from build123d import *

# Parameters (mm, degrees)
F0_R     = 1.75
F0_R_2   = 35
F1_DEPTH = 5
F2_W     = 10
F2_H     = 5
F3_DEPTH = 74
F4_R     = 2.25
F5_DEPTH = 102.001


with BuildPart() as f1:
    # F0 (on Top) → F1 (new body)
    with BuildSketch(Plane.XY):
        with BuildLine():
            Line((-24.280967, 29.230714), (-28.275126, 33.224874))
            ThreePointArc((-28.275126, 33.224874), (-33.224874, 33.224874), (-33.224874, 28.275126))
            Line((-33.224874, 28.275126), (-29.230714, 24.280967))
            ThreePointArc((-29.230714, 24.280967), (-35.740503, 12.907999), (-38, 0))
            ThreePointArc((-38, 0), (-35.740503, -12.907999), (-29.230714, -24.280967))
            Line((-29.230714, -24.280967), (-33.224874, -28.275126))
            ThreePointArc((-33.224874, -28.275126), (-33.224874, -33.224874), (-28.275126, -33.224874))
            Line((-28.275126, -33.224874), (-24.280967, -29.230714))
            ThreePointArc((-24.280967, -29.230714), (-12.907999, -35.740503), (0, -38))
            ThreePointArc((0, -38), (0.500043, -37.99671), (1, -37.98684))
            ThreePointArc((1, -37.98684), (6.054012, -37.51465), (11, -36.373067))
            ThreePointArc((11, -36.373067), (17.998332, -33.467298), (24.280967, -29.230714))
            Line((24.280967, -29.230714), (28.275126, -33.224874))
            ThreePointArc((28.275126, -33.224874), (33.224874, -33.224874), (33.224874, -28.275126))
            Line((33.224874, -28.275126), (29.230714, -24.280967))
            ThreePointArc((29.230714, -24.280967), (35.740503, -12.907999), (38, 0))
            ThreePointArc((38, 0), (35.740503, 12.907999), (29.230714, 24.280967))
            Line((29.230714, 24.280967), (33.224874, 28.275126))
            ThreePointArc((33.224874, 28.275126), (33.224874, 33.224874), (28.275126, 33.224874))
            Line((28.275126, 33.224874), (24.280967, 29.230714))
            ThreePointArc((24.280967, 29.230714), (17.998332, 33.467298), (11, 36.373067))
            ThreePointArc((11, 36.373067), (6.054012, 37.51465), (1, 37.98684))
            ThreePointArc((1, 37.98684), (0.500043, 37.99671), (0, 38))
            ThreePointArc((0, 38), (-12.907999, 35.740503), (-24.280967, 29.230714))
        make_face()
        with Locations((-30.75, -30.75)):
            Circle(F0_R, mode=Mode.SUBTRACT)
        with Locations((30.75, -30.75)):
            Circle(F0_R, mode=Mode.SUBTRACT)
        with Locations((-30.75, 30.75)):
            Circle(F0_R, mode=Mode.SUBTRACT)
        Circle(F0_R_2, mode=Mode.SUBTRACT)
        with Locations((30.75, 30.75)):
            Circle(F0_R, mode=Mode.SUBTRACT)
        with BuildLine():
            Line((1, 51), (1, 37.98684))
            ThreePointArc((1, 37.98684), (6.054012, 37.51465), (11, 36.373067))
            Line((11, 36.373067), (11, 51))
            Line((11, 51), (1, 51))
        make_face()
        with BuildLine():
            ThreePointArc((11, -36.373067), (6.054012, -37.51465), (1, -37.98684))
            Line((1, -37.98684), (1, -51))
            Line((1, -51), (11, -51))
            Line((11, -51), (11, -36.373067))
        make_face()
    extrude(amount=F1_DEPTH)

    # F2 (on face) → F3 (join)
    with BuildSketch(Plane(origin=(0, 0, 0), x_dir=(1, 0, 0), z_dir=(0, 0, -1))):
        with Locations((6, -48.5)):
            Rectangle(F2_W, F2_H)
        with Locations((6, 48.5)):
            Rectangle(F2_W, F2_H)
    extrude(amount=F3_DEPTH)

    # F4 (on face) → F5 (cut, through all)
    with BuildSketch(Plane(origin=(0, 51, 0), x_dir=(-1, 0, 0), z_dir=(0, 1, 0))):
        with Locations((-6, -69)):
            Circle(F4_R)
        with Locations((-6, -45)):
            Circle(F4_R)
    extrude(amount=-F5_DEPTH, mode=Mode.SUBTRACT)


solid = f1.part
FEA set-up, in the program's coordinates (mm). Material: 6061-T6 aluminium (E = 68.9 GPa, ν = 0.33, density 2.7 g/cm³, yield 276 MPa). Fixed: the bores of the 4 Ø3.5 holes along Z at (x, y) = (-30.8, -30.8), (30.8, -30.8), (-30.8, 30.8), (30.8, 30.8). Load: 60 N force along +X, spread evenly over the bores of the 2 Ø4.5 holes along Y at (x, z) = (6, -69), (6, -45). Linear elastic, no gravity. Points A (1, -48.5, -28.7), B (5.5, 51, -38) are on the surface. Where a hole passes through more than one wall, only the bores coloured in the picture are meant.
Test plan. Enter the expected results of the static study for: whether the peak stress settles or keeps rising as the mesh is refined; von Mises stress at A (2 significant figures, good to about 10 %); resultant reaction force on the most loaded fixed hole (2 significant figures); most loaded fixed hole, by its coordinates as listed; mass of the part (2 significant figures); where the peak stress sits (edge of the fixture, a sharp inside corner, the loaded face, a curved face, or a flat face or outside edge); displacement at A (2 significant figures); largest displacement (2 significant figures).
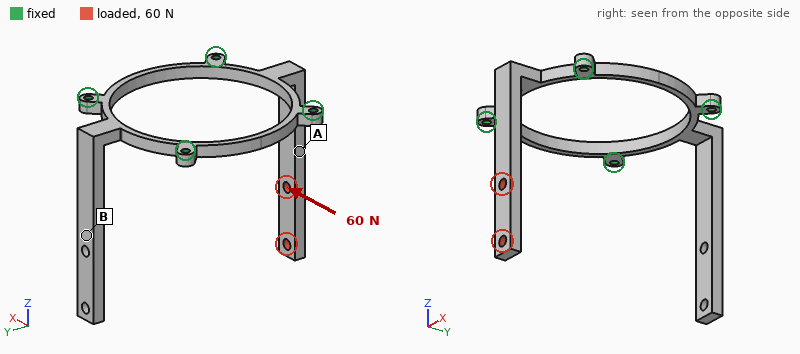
keeps rising
20 MPa
110 N
(-30.8, -30.8)
35 g
a sharp inside corner
0.40 mm
1.1 mm
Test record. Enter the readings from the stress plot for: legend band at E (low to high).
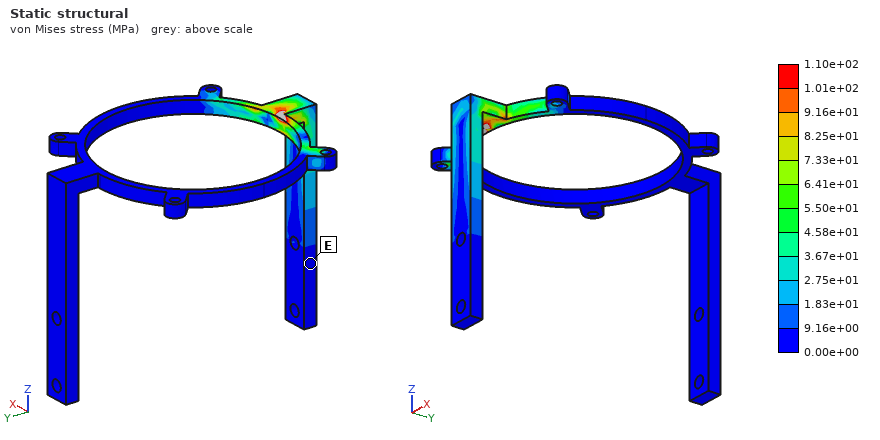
0.00e+00 to 9.16e+00 MPa
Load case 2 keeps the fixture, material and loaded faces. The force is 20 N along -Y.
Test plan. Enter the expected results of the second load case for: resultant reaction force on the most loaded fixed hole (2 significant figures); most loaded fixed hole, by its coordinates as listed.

23 N
(30.8, -30.8)
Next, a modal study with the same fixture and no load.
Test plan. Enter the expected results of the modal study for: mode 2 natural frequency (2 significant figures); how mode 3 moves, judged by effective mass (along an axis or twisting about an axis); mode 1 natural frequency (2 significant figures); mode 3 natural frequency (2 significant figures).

290 Hz
along X
290 Hz
620 Hz
